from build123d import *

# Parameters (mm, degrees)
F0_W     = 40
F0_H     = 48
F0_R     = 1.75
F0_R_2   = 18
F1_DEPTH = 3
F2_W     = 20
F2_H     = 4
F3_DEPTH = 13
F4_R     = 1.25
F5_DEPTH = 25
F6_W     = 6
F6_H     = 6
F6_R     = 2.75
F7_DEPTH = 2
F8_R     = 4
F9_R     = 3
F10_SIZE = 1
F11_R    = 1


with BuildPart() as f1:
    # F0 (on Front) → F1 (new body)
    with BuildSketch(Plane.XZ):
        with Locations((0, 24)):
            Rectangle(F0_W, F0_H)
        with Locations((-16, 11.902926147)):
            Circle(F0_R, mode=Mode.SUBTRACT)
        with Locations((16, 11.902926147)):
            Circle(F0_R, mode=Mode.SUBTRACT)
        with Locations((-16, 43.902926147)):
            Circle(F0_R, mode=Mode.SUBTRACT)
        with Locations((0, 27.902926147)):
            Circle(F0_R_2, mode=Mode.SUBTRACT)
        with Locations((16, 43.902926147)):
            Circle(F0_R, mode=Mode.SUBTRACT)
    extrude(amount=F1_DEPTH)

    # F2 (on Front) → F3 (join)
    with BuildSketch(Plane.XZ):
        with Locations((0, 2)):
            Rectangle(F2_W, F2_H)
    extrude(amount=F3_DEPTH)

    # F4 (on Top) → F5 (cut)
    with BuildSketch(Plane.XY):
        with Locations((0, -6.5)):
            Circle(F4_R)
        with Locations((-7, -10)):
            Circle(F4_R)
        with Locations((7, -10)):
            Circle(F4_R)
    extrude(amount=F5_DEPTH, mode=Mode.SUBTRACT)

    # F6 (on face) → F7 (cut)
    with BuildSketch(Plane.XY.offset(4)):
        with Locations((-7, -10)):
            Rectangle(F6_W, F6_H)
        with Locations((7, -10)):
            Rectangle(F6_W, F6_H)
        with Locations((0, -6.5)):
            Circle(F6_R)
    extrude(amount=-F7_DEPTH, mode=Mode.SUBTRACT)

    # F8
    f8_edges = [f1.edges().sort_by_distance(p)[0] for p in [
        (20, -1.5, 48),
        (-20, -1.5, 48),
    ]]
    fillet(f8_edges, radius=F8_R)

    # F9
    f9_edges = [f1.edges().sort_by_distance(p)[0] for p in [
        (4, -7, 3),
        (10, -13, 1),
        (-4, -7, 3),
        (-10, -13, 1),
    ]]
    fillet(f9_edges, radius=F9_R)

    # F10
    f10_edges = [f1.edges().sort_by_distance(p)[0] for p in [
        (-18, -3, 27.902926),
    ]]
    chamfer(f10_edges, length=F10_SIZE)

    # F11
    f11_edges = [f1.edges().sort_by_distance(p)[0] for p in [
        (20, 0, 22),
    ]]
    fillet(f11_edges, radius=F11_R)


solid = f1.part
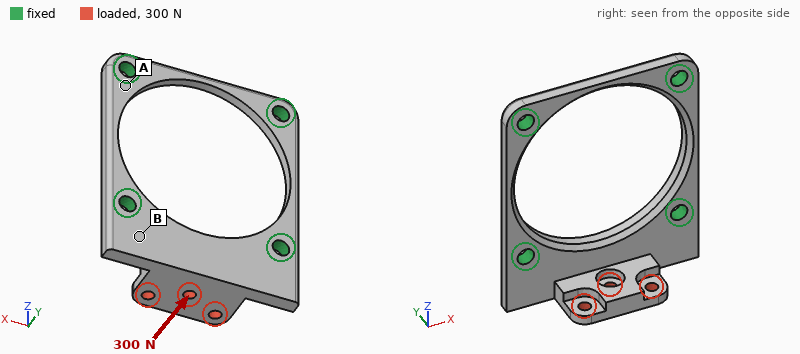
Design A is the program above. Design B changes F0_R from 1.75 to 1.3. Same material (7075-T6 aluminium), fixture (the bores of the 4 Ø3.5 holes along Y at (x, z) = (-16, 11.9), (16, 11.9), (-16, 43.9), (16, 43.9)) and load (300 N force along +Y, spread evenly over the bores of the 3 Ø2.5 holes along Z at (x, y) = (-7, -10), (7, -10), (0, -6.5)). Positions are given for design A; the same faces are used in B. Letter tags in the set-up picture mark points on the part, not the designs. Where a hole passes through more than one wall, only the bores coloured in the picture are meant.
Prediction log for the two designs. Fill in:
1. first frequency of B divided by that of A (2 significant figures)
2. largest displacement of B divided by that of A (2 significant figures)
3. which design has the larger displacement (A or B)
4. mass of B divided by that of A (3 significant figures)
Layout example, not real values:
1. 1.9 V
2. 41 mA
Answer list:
1. 0.93
2. 1.1
3. B
4. 1.02
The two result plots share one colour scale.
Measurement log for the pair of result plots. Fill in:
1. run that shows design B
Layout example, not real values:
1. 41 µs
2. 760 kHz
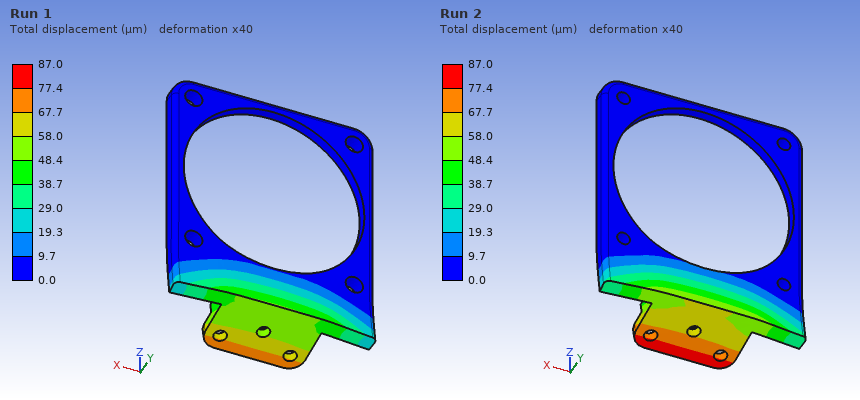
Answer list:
1. Run 2
